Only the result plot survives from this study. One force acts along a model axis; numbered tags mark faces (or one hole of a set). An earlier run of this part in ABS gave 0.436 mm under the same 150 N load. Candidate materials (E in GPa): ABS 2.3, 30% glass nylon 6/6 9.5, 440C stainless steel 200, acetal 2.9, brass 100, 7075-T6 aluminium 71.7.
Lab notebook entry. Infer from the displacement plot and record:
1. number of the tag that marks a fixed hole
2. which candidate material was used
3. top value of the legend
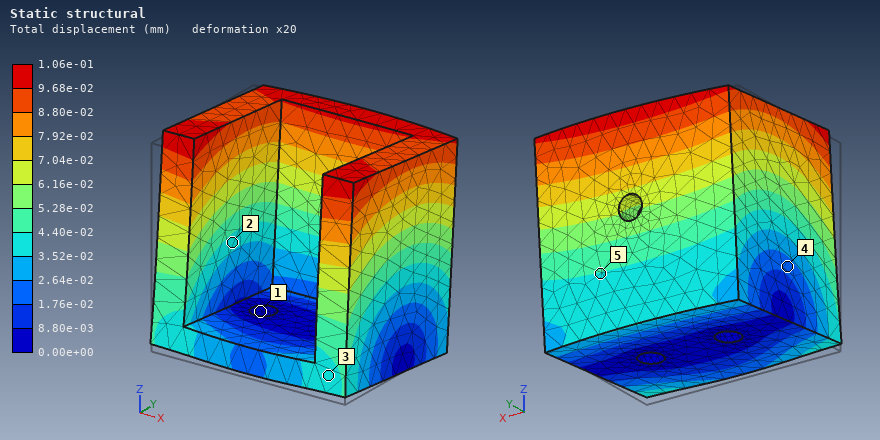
1
30% glass nylon 6/6
1.06e-01 mm
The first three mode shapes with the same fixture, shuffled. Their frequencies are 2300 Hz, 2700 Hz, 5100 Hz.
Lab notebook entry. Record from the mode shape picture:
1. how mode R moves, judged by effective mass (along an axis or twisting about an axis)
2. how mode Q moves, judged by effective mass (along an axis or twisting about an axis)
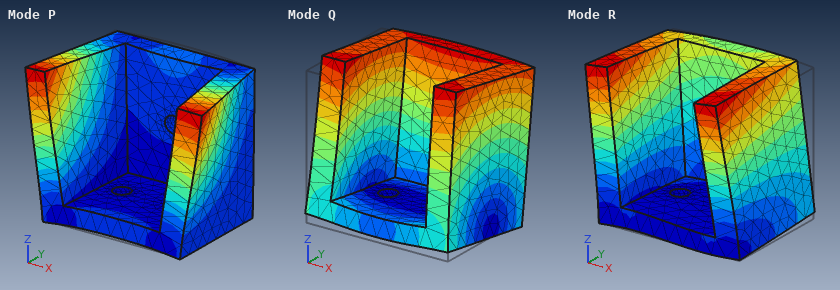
along X
along Y
